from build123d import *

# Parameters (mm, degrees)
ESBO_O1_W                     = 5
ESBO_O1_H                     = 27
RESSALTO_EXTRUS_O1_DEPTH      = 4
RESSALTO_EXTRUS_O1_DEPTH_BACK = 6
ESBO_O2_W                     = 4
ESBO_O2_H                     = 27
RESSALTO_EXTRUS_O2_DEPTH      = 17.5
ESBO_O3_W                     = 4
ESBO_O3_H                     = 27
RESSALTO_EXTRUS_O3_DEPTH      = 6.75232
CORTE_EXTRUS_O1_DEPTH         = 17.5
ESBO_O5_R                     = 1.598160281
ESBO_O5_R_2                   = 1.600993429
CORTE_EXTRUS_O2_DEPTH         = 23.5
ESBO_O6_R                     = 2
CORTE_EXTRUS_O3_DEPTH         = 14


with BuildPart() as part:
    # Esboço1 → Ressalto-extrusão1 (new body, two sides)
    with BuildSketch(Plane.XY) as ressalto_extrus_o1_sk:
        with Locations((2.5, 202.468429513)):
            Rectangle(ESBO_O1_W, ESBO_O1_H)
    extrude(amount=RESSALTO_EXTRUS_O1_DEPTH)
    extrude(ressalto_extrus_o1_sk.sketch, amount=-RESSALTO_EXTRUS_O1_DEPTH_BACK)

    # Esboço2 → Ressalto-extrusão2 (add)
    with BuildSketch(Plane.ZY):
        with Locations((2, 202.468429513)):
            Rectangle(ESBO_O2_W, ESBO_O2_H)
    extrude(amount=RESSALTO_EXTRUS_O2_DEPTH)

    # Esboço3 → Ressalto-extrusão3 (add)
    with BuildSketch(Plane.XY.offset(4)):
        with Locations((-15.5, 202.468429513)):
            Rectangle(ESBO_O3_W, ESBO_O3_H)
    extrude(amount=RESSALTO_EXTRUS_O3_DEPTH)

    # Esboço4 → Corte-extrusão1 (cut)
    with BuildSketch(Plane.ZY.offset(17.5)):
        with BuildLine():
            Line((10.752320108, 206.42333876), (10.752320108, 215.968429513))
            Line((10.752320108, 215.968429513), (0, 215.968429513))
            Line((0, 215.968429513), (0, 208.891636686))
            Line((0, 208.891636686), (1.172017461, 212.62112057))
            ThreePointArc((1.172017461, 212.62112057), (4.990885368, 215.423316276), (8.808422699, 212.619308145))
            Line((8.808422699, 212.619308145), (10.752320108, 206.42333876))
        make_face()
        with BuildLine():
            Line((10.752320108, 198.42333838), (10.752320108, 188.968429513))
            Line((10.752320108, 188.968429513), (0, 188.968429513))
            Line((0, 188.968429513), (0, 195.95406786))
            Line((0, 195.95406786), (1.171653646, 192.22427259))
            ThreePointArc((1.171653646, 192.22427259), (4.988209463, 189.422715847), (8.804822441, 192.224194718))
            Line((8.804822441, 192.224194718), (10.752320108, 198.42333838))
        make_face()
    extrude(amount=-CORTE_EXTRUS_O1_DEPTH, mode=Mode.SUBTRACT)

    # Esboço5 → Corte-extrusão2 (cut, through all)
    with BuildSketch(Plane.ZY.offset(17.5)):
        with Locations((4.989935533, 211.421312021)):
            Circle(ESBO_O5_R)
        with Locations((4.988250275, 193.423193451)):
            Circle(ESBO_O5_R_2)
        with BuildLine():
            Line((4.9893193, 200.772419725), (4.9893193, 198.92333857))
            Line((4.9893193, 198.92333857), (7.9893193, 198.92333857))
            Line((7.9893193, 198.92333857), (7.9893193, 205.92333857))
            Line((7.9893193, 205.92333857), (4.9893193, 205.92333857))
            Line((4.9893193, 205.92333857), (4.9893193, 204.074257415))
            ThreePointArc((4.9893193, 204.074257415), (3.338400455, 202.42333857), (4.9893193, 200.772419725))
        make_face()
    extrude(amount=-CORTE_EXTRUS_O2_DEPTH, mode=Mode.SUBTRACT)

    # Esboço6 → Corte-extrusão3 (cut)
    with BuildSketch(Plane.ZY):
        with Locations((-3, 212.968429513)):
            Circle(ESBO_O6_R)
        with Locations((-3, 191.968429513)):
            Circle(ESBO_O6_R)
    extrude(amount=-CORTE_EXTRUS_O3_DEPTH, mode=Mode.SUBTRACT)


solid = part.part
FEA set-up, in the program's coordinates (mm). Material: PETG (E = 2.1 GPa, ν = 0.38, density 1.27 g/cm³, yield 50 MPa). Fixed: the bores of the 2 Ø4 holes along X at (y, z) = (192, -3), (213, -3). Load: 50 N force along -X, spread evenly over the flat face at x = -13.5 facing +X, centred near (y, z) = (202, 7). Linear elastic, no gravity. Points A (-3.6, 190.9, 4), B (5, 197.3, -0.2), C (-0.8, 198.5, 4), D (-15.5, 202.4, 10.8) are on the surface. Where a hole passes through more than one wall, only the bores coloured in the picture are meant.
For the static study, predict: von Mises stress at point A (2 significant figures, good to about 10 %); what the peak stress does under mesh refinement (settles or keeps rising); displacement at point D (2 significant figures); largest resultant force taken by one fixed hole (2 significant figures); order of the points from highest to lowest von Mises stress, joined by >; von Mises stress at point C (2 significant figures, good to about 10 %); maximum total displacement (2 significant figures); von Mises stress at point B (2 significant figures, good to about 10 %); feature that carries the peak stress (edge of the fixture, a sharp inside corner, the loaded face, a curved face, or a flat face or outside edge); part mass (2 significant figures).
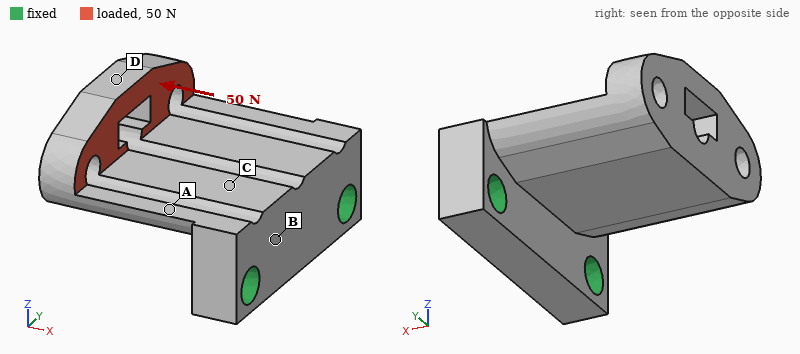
6.0 MPa
keeps rising
0.35 mm
25 N
A > C > B > D
4.6 MPa
0.39 mm
2.0 MPa
edge of the fixture
4.0 g
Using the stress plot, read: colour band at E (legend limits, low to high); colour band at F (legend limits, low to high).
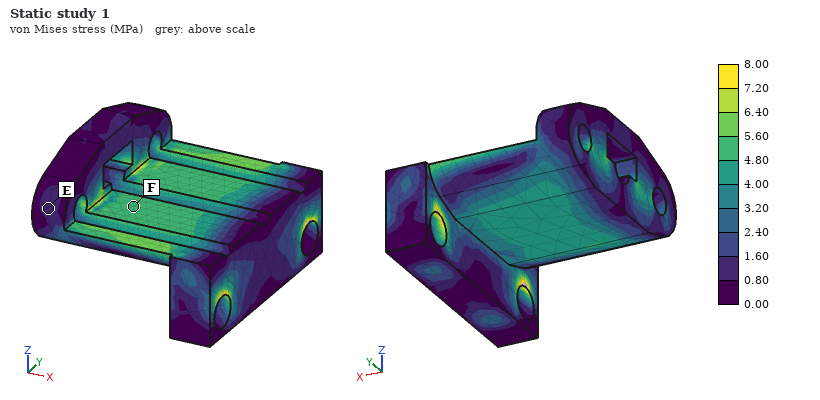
0.80 to 1.60 MPa
4.80 to 5.60 MPa
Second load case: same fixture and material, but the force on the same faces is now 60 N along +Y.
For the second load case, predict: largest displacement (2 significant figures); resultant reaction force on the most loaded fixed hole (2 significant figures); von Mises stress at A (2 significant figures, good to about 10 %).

0.22 mm
63 N
2.8 MPa
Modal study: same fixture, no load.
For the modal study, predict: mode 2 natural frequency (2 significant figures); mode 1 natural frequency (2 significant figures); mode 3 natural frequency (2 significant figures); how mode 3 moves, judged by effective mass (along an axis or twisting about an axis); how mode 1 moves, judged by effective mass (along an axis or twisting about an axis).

2700 Hz
1300 Hz
4400 Hz
along Y
along Z
